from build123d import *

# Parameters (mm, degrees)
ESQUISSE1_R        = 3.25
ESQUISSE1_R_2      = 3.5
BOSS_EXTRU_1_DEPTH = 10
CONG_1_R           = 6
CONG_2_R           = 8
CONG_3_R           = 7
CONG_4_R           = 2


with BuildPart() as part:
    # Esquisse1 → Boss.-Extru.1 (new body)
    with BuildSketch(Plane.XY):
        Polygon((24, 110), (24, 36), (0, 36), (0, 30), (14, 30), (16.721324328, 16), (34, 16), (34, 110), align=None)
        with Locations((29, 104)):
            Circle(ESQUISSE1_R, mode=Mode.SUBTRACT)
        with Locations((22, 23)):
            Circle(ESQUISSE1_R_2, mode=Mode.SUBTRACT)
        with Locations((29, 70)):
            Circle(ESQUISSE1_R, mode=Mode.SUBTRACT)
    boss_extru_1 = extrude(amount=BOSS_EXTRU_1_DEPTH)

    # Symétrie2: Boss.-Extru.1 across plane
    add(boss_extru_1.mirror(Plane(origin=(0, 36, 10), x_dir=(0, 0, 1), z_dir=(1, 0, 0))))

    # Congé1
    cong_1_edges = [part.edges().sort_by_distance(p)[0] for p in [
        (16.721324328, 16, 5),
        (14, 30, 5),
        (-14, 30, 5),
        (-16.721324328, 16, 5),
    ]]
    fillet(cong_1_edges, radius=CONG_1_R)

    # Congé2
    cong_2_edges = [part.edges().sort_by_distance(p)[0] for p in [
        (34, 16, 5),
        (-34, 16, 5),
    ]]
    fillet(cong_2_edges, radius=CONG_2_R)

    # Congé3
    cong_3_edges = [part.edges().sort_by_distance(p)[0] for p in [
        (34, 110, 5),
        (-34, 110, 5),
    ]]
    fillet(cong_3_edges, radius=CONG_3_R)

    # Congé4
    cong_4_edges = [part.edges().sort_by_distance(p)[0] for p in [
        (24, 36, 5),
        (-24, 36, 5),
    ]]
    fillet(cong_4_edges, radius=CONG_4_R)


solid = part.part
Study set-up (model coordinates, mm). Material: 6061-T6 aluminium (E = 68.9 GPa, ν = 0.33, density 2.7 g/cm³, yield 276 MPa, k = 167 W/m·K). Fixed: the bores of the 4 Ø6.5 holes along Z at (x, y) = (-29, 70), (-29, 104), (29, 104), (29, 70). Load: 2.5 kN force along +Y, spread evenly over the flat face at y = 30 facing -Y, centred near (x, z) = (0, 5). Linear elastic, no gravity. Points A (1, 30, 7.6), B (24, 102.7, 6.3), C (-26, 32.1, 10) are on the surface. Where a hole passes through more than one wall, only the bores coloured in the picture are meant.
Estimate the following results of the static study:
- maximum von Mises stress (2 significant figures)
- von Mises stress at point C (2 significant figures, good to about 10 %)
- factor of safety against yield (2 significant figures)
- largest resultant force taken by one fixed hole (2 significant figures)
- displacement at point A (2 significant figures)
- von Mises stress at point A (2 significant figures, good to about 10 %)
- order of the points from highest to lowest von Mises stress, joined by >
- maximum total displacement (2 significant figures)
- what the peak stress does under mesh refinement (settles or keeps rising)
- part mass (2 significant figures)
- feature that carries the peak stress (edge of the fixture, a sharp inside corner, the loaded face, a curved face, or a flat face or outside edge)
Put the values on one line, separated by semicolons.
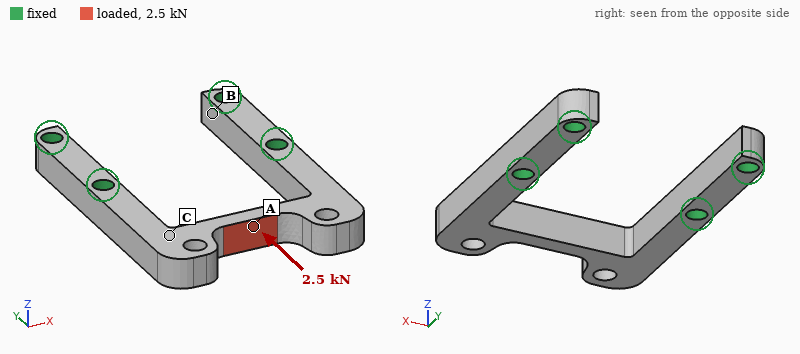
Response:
230 MPa; 43 MPa; 1.2; 1.5 kN; 0.14 mm; 160 MPa; A > C > B; 0.14 mm; settles; 58 g; a curved face
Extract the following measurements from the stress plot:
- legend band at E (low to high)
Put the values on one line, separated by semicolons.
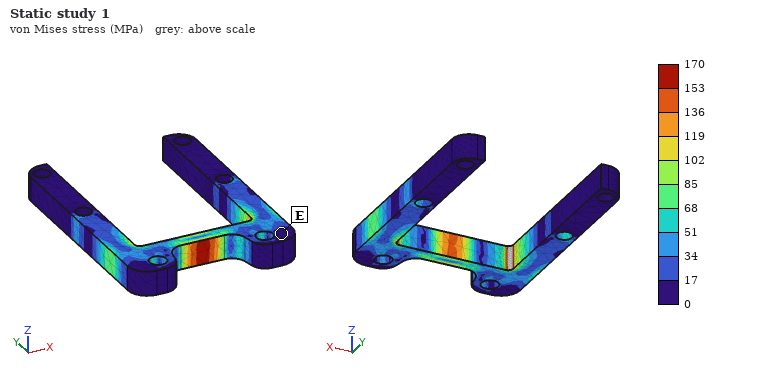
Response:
0 to 17 MPa
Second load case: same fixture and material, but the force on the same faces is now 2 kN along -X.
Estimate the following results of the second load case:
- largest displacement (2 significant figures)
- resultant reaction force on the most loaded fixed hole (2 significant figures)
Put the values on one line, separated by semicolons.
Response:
0.15 mm; 1.2 kN
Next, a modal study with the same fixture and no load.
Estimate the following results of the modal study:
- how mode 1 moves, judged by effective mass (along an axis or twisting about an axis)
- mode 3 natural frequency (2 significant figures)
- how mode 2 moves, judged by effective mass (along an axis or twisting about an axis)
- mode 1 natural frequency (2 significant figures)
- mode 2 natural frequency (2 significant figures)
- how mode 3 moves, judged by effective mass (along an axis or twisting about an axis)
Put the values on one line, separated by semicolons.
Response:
along Z; 3600 Hz; twisting about Y; 2300 Hz; 3400 Hz; along X
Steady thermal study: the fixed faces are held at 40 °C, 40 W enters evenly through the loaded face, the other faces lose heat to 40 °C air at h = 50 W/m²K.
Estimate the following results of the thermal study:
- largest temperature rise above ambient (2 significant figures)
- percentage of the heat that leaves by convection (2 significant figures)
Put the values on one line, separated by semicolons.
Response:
66 K; 22 %
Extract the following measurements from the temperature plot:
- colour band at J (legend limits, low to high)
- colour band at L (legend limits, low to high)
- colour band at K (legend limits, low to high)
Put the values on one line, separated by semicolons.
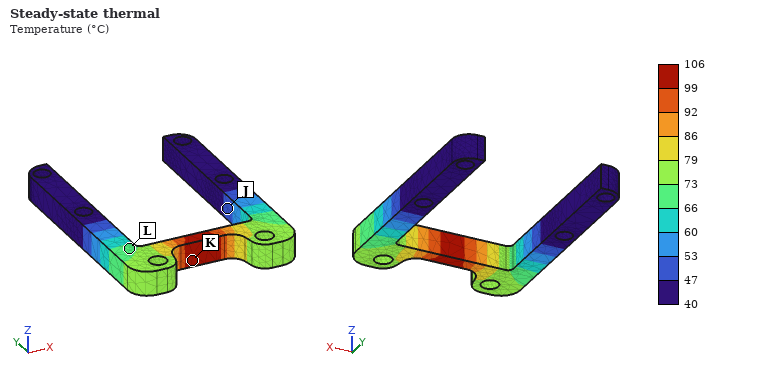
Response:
47 to 53 °C; 66 to 73 °C; 99 to 106 °C
